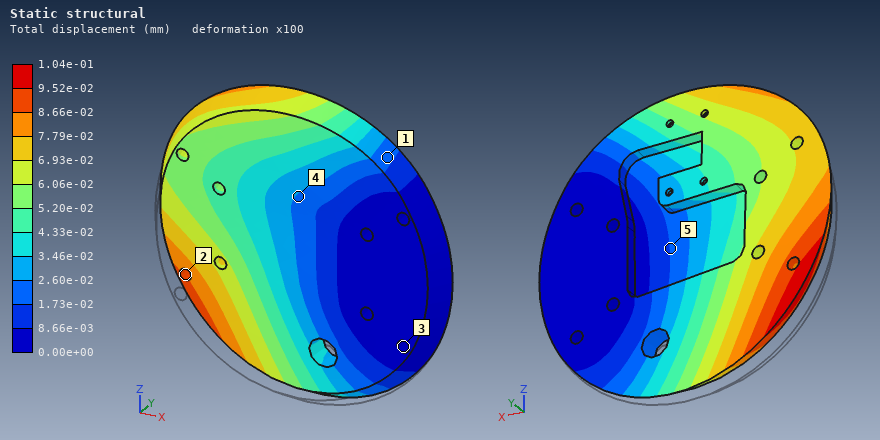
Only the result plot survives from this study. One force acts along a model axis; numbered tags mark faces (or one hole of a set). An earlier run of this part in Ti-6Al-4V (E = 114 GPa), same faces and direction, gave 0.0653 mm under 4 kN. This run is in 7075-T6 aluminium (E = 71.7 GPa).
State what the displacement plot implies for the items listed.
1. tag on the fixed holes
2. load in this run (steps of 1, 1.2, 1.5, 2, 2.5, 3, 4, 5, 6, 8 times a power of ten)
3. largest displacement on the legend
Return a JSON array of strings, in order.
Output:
["3", "4 kN", "1.04e-01 mm"]
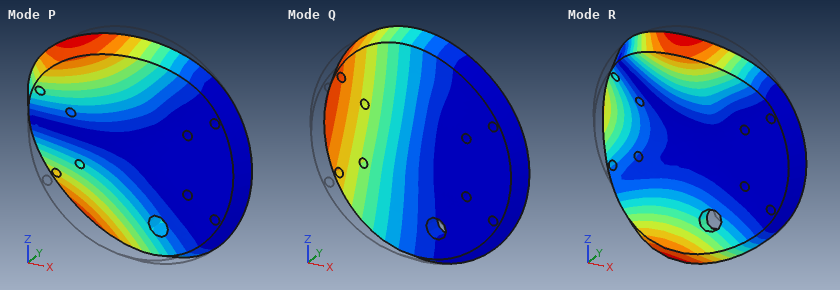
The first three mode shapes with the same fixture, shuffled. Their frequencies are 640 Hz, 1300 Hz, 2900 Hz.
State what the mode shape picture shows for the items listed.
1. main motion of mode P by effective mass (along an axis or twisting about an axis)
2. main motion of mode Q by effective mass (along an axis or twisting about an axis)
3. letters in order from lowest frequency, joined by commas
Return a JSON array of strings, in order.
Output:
["twisting about X", "along Y", "Q, P, R"]
